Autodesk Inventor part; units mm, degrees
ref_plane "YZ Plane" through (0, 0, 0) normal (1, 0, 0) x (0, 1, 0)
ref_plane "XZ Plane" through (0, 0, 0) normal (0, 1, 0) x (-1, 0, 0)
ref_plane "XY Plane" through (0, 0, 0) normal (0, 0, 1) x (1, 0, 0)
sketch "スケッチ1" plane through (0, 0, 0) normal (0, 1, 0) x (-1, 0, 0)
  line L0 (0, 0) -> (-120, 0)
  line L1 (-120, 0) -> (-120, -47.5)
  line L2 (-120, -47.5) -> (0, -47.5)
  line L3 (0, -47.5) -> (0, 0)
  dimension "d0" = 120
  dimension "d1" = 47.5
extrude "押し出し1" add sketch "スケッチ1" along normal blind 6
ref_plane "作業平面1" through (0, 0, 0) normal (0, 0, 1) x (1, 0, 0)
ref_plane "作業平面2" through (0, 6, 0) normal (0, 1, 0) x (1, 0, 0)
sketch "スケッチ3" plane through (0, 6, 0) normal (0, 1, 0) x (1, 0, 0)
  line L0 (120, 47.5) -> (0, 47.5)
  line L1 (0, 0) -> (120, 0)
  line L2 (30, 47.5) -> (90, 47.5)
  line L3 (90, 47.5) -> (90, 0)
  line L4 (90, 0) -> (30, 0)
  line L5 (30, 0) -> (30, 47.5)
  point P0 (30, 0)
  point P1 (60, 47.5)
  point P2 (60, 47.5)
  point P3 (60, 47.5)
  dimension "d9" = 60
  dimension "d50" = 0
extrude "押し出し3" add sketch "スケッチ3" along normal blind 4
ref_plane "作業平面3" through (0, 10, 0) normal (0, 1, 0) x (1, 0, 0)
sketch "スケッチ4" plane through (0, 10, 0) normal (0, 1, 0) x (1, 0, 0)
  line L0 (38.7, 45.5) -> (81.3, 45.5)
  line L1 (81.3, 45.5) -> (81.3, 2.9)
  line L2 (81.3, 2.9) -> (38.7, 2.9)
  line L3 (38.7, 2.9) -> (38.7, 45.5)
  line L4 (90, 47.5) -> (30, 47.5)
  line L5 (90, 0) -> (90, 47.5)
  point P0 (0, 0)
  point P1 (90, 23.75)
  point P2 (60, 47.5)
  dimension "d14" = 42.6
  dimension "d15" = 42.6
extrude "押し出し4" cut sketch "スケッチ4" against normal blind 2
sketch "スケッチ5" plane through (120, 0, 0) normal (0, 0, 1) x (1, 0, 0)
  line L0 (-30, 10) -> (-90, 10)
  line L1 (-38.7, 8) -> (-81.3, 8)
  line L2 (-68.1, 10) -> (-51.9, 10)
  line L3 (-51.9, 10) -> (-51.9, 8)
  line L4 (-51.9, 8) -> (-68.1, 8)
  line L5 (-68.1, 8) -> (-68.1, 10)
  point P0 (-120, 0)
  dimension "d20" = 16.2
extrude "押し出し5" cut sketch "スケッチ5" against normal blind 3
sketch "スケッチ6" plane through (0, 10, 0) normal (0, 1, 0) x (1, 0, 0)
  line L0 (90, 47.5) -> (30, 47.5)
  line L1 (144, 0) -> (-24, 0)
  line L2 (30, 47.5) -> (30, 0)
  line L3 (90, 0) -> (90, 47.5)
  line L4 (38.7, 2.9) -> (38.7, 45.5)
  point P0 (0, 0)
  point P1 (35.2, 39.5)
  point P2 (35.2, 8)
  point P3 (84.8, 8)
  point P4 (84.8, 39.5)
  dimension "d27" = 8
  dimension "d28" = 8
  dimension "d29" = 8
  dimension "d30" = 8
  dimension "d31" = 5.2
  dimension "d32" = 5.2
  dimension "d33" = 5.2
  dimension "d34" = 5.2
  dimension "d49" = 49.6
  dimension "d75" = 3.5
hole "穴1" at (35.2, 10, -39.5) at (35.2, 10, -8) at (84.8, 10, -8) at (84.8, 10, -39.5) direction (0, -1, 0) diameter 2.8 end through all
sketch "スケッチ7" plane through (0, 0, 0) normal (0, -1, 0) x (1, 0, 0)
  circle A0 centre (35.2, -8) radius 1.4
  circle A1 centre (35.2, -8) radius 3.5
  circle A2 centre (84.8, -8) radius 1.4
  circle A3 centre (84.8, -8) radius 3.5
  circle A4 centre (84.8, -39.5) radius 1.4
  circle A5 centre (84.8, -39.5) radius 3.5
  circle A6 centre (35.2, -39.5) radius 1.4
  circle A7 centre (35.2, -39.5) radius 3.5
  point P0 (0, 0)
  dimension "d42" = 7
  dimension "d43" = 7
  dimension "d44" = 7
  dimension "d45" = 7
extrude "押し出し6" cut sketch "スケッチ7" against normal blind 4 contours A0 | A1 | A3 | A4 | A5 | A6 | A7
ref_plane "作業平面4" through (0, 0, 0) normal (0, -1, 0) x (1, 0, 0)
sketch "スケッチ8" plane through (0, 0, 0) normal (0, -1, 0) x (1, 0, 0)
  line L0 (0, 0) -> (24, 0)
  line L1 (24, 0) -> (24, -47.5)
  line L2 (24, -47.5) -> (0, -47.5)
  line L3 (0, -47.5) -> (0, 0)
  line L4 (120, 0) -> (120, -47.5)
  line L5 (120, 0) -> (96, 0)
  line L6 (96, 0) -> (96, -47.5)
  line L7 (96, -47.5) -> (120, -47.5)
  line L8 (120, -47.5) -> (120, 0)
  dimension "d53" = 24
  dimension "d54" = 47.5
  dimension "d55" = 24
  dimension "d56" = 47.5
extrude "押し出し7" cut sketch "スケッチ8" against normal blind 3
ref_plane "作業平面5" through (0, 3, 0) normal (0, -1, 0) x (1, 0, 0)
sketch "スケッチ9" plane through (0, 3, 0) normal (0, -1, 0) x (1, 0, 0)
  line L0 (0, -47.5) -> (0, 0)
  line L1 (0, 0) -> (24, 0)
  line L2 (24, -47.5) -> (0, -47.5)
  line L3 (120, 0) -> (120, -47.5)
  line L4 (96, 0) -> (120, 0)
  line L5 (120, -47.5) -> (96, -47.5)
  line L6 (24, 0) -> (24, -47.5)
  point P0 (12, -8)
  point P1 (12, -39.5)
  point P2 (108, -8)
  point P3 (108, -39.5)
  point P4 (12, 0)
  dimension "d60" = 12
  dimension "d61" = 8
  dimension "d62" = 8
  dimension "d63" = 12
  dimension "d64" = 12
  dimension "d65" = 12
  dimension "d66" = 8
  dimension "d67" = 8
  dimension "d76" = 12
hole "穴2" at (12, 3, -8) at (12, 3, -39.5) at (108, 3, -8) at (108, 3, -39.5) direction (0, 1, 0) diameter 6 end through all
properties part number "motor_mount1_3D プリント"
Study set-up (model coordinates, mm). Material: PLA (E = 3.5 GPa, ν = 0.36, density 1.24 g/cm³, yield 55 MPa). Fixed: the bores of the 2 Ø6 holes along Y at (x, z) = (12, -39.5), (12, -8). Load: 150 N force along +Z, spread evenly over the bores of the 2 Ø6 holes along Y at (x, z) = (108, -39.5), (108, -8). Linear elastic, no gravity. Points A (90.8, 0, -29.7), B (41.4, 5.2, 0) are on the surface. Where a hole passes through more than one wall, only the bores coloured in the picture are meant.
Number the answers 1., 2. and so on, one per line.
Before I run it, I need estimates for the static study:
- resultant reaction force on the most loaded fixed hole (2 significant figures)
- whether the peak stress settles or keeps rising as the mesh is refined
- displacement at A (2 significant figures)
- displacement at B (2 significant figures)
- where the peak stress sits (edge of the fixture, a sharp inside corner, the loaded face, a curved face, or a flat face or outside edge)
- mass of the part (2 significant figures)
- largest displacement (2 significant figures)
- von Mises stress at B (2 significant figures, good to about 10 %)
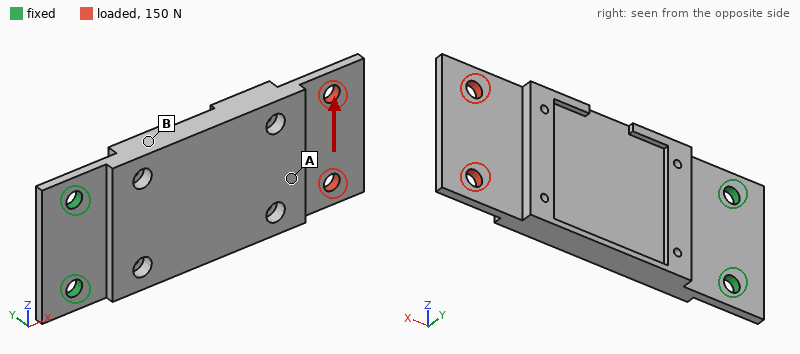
1. 430 N
2. keeps rising
3. 0.28 mm
4. 0.12 mm
5. edge of the fixture
6. 42 g
7. 0.46 mm
8. 3.4 MPa
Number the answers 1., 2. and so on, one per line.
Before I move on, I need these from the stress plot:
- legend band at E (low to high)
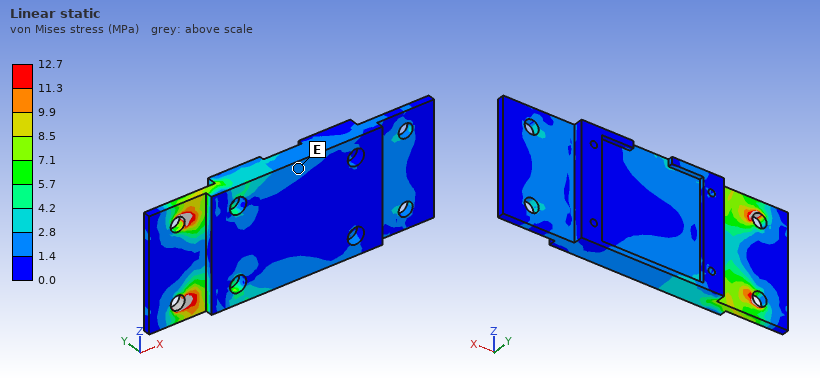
1. 1.4 to 2.8 MPa
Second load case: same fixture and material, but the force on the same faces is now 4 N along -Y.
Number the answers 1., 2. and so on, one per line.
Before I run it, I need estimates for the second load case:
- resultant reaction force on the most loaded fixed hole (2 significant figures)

1. 2.0 N
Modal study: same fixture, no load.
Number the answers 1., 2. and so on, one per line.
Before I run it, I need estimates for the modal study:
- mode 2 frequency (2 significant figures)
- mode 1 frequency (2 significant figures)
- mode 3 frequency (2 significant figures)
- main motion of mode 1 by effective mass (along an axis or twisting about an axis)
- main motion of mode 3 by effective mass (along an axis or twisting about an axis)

1. 700 Hz
2. 86 Hz
3. 900 Hz
4. along Y
5. along Z
